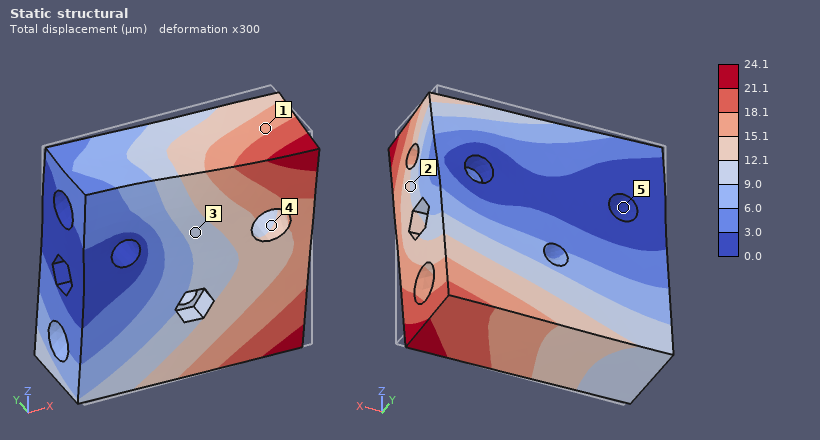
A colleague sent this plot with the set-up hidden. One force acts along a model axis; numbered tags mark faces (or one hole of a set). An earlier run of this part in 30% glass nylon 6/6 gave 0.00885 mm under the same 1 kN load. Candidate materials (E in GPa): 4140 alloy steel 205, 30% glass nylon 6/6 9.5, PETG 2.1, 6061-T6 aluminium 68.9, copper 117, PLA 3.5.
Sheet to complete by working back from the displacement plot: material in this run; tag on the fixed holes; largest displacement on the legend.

PLA
5
24.1 µm
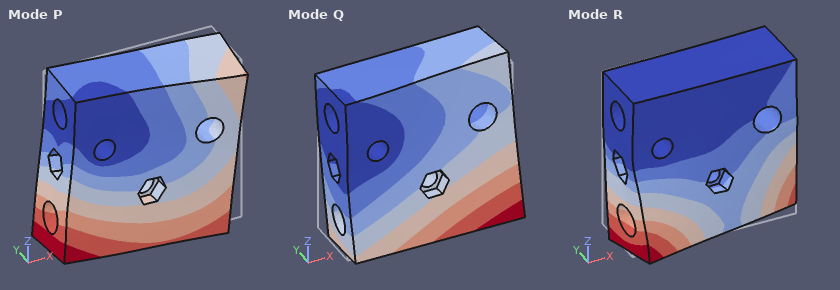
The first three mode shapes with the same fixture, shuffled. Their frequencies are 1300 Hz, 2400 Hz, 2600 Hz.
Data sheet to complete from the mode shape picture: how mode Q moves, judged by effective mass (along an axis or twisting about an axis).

along Y
